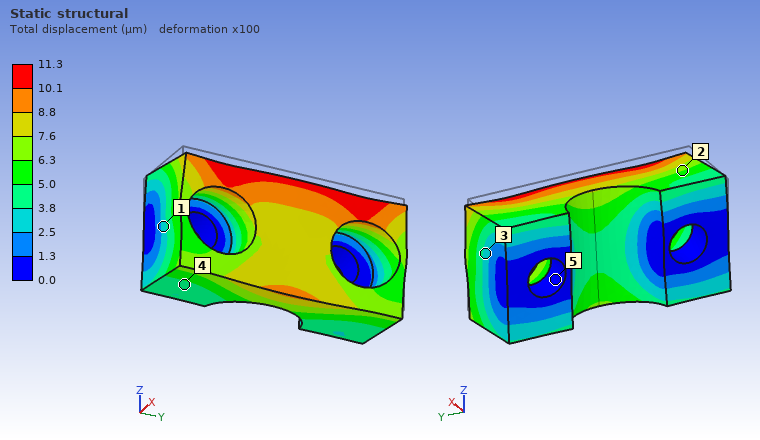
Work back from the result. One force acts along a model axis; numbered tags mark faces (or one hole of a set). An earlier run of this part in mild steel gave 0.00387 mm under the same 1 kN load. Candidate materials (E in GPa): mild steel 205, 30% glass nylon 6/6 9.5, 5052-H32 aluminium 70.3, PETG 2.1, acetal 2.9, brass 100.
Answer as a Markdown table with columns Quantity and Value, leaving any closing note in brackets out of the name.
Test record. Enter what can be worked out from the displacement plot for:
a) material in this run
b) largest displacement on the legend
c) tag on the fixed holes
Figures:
| Quantity | Value |
|---|---|
| material in this run | 5052-H32 aluminium |
| largest displacement on the legend | 11.3 µm |
| tag on the fixed holes | 5 |
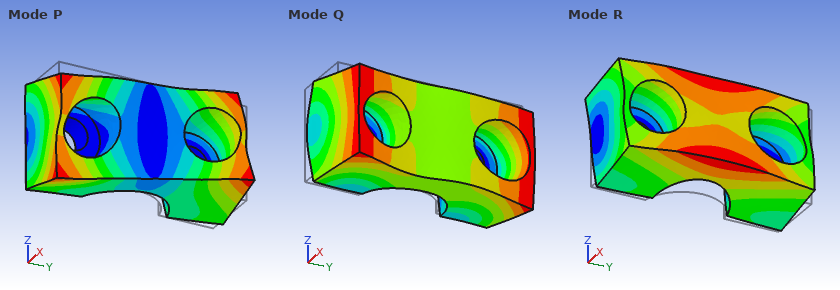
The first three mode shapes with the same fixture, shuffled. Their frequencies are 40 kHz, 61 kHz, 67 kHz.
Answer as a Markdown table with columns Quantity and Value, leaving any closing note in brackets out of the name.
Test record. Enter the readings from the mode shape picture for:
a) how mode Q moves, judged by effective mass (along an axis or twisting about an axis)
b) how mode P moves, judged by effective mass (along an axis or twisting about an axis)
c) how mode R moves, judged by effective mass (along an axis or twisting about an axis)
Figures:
| Quantity | Value |
|---|---|
| how mode Q moves, judged by effective mass | along Y |
| how mode P moves, judged by effective mass | twisting about X |
| how mode R moves, judged by effective mass | along Z |
